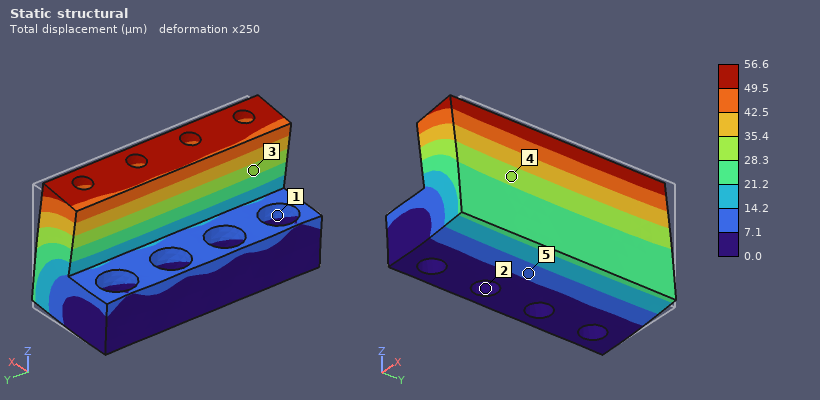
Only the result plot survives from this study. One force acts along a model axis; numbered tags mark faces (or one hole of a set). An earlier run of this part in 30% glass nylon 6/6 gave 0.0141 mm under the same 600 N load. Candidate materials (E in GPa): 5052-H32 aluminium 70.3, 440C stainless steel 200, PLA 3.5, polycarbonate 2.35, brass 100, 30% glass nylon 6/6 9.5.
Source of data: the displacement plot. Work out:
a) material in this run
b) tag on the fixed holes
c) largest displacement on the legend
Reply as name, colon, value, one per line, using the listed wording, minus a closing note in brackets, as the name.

material in this run: polycarbonate
tag on the fixed holes: 2
largest displacement on the legend: 56.6 µm
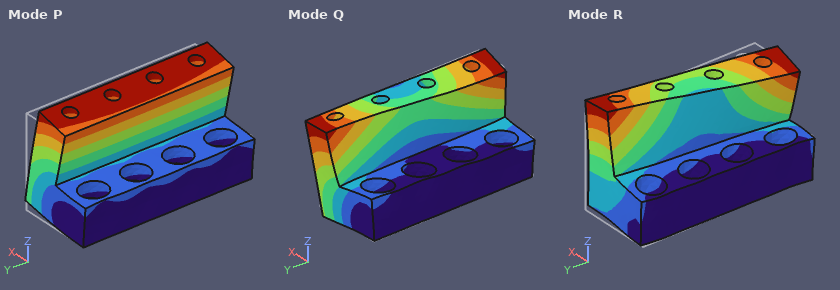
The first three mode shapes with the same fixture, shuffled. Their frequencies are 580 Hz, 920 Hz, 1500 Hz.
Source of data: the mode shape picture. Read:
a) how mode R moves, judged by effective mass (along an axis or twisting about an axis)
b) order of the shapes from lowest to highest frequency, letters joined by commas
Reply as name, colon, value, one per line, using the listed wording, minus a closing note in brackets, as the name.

how mode R moves, judged by effective mass: along Y
order of the shapes from lowest to highest frequency, letters joined by commas: P, Q, R
